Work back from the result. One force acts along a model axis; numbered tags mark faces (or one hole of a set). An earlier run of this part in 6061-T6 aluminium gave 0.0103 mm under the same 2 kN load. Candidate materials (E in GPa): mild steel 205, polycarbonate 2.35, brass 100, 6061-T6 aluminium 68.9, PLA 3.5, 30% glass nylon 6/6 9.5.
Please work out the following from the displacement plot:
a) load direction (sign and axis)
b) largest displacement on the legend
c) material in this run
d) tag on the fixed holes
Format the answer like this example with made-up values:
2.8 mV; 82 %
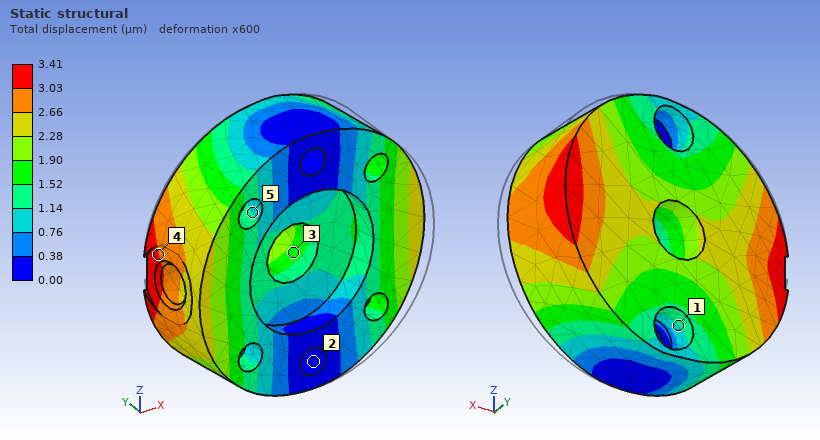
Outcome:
-X; 3.41 µm; mild steel; 2
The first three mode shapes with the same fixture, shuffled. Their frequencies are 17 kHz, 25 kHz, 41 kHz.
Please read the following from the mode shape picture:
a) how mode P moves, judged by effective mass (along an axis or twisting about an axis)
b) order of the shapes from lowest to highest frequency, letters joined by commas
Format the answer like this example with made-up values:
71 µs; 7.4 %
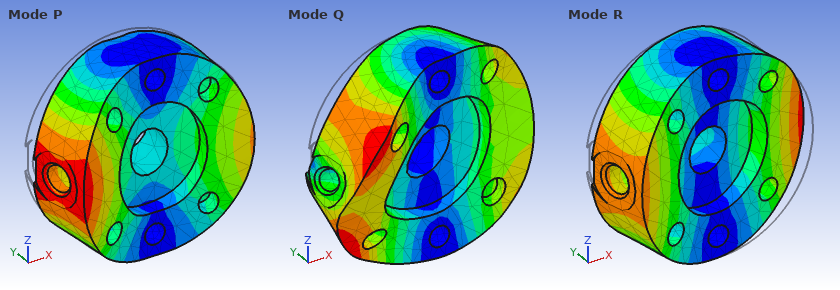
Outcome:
along Y; R, P, Q
